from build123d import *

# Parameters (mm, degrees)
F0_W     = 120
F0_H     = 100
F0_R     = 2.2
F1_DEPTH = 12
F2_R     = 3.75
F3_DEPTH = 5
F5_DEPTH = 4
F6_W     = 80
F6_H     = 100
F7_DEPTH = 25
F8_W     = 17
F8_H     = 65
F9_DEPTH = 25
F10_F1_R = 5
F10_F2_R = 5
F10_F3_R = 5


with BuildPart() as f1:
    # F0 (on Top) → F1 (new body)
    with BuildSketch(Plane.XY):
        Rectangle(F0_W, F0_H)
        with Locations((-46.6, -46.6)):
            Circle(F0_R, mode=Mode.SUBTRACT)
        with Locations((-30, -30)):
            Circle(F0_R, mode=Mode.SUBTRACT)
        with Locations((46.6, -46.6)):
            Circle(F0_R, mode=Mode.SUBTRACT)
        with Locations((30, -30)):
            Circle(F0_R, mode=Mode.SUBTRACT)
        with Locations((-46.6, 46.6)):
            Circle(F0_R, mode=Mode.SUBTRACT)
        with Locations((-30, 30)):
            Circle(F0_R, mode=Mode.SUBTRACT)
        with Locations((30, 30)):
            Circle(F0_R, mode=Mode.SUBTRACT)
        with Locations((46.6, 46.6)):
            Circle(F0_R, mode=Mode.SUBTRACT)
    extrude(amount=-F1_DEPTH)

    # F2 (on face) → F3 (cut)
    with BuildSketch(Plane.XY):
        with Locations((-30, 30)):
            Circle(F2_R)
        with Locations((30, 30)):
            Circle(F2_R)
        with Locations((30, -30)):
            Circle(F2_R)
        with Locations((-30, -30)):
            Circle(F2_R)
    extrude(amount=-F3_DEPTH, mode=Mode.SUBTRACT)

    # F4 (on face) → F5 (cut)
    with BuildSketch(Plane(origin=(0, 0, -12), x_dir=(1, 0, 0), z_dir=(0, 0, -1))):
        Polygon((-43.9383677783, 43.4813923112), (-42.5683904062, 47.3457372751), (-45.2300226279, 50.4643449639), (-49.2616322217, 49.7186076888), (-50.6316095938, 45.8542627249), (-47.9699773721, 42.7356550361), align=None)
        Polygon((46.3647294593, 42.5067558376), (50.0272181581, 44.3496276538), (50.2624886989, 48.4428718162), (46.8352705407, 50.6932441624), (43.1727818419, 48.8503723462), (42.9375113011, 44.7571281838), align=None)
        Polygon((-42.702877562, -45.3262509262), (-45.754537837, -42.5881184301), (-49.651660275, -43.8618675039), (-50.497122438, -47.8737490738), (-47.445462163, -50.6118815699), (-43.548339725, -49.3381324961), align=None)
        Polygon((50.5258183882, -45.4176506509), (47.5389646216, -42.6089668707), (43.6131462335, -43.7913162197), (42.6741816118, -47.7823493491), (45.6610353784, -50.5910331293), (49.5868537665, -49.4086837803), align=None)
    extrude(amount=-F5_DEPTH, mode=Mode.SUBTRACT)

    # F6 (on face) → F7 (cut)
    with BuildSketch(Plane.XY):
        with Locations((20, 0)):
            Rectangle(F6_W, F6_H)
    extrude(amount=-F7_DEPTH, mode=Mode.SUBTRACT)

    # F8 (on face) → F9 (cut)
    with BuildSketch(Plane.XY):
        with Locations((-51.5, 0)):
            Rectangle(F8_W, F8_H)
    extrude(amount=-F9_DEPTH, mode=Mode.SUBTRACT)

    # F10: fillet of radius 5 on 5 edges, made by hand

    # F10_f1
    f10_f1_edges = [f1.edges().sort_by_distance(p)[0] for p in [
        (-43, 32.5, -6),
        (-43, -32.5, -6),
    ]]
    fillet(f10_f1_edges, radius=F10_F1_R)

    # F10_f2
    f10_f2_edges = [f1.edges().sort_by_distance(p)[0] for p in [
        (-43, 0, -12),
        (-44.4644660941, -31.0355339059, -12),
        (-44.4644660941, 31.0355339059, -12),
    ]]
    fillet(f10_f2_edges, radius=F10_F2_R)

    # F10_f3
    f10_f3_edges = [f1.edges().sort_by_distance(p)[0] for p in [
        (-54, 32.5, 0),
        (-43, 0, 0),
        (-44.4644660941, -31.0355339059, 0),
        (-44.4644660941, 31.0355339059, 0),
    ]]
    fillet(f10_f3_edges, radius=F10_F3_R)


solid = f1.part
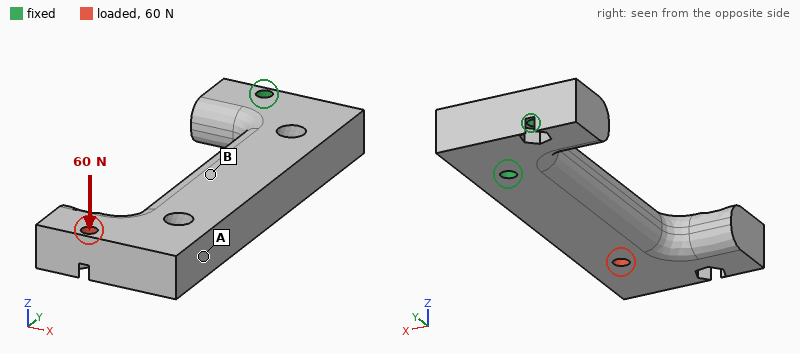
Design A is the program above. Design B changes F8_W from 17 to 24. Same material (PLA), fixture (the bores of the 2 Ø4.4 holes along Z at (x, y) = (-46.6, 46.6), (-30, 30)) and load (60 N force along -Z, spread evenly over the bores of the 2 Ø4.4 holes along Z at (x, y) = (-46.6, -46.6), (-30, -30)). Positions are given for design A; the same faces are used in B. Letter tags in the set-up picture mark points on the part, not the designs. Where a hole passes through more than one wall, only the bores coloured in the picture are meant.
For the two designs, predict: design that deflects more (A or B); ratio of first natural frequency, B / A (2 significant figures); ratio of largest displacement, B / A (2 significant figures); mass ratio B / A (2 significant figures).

B
0.94
1.2
0.91
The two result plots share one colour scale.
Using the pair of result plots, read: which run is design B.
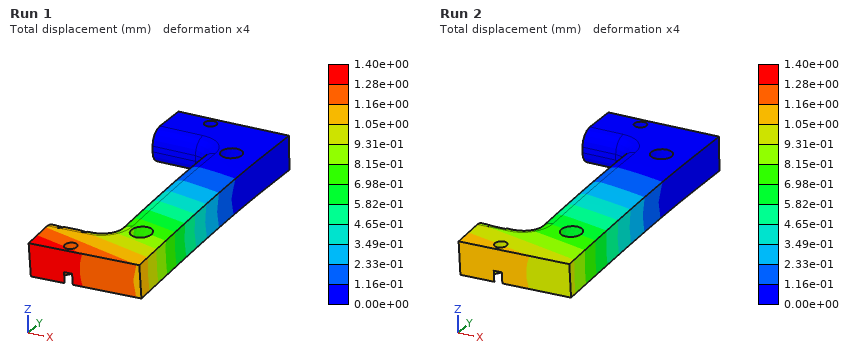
Run 1
